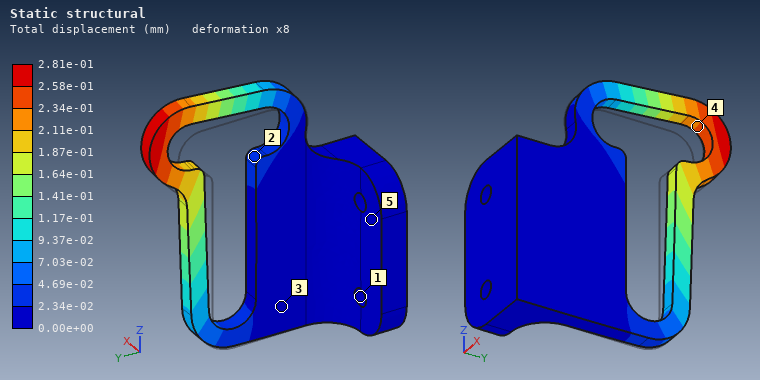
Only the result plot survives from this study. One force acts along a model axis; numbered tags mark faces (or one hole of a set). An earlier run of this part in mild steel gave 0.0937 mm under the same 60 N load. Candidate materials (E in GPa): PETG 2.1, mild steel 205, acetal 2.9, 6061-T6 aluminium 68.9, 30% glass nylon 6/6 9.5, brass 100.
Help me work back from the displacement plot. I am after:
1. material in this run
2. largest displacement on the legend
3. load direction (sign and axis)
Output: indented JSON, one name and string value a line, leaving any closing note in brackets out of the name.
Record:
{
  "material in this run": "6061-T6 aluminium",
  "largest displacement on the legend": "2.81e-01 mm",
  "load direction": "+X"
}
